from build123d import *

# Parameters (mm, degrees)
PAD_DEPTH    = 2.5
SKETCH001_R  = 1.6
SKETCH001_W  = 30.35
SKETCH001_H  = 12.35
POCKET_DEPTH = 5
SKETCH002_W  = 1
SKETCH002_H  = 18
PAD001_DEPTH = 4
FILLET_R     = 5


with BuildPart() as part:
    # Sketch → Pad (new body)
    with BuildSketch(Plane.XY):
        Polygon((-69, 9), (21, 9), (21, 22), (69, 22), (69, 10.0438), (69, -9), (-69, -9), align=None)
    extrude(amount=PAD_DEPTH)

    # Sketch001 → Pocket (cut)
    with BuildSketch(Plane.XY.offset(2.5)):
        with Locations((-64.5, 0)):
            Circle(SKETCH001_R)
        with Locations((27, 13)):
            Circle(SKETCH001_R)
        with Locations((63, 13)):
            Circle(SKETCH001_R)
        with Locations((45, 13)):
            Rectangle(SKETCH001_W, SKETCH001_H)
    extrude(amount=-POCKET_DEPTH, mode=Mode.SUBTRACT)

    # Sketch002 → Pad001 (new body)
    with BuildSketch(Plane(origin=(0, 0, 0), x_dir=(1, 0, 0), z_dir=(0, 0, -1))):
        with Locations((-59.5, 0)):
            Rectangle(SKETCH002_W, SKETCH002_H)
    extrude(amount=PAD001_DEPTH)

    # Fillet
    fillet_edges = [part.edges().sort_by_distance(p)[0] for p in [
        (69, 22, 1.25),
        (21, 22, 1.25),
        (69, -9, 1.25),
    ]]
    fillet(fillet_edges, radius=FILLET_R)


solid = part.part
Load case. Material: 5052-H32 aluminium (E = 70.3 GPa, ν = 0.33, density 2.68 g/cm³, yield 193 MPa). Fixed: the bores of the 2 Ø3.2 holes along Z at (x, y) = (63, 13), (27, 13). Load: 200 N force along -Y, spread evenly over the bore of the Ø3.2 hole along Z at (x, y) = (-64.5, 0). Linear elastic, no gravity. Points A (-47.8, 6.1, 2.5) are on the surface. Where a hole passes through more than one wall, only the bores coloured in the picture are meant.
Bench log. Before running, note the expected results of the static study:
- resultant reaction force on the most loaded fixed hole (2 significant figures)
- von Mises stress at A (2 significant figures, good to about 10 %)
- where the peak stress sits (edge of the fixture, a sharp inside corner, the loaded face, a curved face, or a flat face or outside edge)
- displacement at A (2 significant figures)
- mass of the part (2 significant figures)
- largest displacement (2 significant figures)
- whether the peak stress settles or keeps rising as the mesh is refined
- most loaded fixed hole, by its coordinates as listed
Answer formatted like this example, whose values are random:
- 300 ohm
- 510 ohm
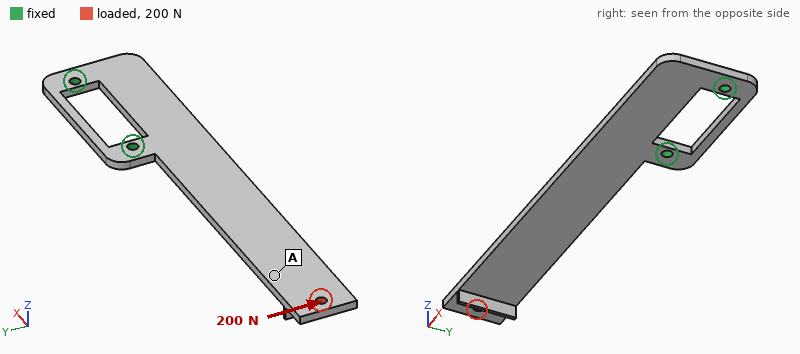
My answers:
- 780 N
- 18 MPa
- a sharp inside corner
- 0.57 mm
- 18 g
- 0.82 mm
- keeps rising
- (27, 13)
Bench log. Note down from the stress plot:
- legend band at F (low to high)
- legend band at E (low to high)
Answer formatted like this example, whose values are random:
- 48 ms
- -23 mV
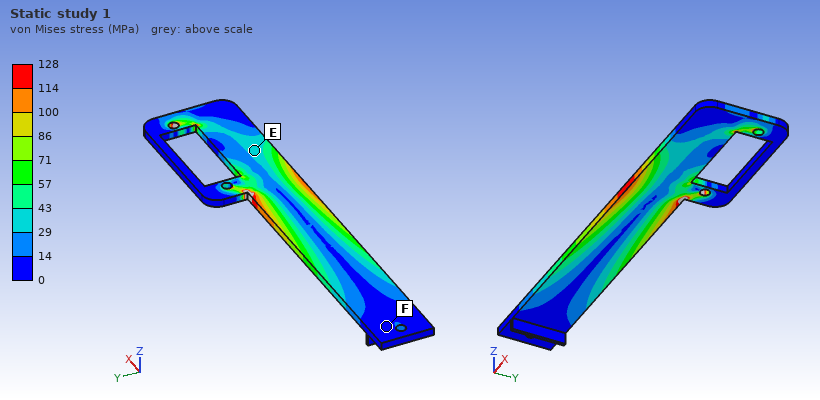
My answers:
- 0 to 14 MPa
- 29 to 43 MPa
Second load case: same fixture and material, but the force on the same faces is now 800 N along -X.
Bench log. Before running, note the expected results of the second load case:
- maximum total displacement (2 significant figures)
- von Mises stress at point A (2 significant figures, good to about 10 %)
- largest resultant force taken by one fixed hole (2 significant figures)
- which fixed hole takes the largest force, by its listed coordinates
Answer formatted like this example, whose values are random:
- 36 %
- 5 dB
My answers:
- 94 µm
- 18 MPa
- 530 N
- (27, 13)
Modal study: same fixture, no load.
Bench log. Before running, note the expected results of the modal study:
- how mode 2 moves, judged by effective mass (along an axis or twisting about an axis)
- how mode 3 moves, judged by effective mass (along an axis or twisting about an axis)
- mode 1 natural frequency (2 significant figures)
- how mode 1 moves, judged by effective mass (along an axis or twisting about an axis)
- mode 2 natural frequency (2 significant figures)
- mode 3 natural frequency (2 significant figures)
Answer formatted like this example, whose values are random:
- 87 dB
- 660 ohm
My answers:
- along Z
- along Y
- 200 Hz
- along Z
- 1200 Hz
- 1400 Hz
